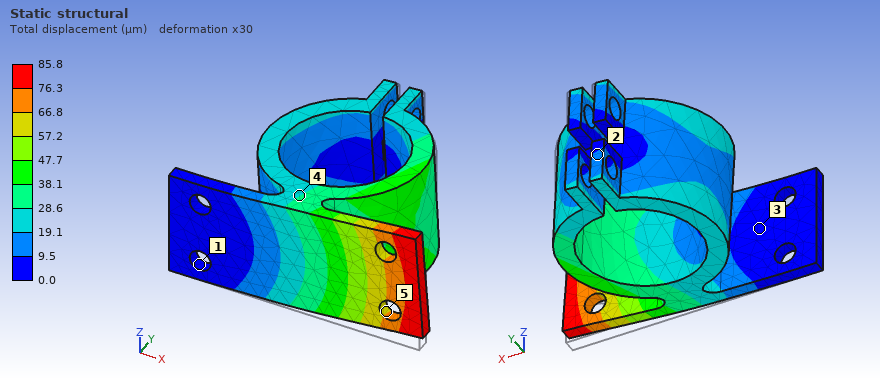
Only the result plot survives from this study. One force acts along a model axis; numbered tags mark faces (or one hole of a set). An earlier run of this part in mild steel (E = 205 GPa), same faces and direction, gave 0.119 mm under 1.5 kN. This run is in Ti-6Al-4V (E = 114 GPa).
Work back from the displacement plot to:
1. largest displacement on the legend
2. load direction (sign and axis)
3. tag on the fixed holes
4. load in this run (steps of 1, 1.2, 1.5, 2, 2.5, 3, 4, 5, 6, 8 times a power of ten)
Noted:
85.8 µm
+Z
1
600 N
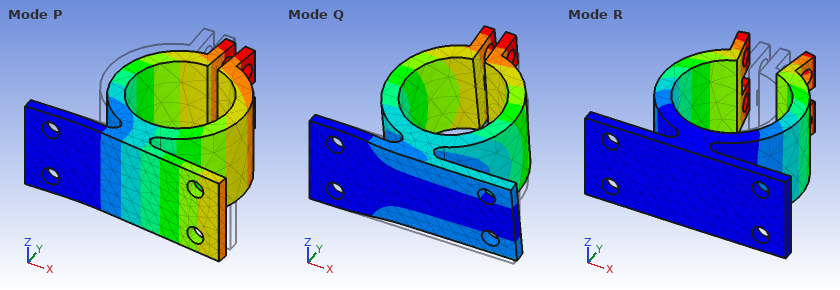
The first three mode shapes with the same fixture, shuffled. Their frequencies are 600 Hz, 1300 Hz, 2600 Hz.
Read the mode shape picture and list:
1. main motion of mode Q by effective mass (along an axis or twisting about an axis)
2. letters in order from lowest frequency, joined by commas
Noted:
along Z
P, Q, R
